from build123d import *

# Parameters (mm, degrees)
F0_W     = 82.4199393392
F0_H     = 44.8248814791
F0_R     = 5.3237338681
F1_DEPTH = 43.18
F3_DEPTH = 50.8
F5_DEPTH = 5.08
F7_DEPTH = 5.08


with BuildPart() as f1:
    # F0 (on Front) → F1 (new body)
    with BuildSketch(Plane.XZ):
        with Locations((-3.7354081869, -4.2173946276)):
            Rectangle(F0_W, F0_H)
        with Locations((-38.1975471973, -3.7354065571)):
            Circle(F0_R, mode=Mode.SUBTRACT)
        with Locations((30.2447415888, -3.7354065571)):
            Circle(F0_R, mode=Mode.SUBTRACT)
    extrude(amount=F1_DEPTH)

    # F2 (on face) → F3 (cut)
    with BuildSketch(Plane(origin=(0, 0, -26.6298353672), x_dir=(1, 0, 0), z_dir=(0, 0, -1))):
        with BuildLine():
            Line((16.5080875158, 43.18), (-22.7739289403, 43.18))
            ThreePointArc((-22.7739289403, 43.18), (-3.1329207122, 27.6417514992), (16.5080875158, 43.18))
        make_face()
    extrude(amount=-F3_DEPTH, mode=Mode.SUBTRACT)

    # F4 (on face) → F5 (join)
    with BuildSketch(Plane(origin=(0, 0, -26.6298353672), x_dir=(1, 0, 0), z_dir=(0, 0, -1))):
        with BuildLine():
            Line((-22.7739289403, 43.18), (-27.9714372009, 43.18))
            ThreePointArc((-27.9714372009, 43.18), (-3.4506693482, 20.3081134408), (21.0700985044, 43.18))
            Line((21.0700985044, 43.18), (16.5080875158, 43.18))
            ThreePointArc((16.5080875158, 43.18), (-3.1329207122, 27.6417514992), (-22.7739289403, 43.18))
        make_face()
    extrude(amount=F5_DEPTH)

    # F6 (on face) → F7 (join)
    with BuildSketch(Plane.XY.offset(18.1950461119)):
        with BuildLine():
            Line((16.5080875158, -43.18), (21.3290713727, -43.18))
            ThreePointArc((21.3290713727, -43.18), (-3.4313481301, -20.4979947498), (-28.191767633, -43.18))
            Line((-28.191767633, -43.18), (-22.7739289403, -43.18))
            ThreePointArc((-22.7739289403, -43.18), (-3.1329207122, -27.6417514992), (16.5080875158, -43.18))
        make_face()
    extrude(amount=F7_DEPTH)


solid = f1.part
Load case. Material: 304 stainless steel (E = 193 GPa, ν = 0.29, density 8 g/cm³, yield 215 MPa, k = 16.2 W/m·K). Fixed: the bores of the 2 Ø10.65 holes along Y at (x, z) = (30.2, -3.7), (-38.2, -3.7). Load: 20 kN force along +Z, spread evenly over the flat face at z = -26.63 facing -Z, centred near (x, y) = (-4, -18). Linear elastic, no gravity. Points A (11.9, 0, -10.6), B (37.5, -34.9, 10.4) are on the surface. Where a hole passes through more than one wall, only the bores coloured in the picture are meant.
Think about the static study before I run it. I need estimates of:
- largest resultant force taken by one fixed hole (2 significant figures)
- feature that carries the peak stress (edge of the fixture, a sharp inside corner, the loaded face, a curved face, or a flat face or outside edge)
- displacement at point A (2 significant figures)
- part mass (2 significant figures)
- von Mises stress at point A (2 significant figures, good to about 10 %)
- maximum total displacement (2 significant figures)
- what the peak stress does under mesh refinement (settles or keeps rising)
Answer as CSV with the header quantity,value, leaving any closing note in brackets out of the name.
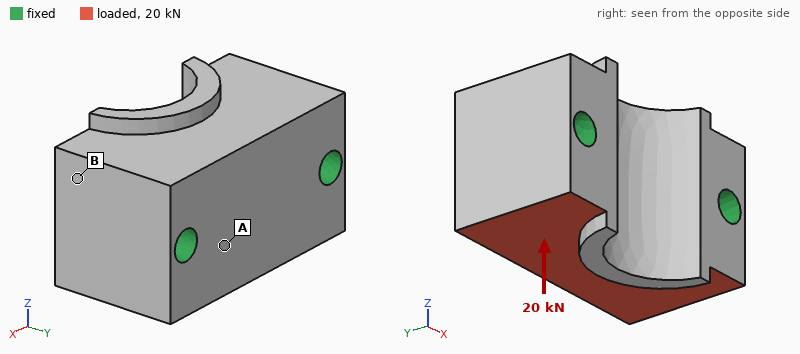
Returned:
quantity,value
largest resultant force taken by one fixed hole,10 kN
feature that carries the peak stress,edge of the fixture
displacement at point A,1.7 µm
part mass,1.1 kg
von Mises stress at point A,7.9 MPa
maximum total displacement,2.8 µm
what the peak stress does under mesh refinement,keeps rising
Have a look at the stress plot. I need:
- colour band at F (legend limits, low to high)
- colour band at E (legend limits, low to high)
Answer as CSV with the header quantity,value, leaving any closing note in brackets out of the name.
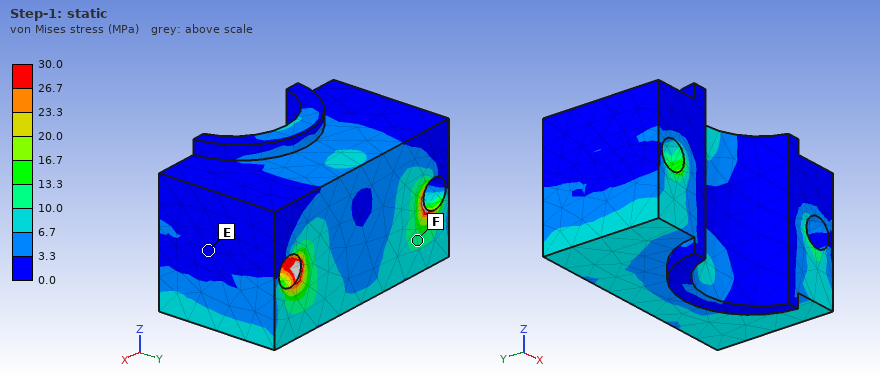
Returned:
quantity,value
colour band at F,10.0 to 13.3 MPa
colour band at E,0.0 to 3.3 MPa
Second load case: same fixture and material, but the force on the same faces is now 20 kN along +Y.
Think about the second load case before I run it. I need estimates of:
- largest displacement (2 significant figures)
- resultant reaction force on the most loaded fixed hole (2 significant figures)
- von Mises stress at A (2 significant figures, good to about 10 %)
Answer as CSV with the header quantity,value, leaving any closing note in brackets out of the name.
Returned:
quantity,value
largest displacement,6.6 µm
resultant reaction force on the most loaded fixed hole,10 kN
von Mises stress at A,11 MPa
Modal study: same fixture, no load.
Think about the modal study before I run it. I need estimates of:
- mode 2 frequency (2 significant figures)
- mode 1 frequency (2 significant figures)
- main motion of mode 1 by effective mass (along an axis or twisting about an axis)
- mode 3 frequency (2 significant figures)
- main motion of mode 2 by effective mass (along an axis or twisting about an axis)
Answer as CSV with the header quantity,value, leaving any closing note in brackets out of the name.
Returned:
quantity,value
mode 2 frequency,18 kHz
mode 1 frequency,17 kHz
main motion of mode 1 by effective mass,along Z
mode 3 frequency,21 kHz
main motion of mode 2 by effective mass,along Y
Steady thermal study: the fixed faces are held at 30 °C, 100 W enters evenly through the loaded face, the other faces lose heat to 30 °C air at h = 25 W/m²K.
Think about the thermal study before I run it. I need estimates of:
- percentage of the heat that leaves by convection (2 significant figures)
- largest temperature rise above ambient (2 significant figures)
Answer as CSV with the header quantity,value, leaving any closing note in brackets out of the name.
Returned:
quantity,value
percentage of the heat that leaves by convection,6.5 %
largest temperature rise above ambient,60 K
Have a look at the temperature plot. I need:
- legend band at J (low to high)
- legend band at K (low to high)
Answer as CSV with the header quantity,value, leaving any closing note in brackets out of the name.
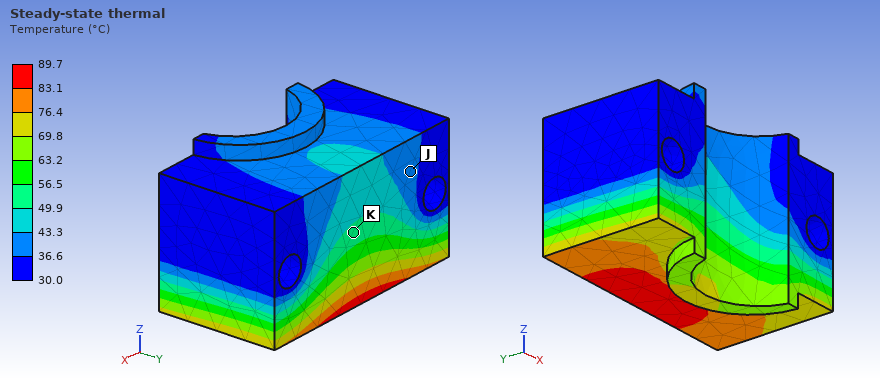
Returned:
quantity,value
legend band at J,36.6 to 43.3 °C
legend band at K,49.9 to 56.5 °C
